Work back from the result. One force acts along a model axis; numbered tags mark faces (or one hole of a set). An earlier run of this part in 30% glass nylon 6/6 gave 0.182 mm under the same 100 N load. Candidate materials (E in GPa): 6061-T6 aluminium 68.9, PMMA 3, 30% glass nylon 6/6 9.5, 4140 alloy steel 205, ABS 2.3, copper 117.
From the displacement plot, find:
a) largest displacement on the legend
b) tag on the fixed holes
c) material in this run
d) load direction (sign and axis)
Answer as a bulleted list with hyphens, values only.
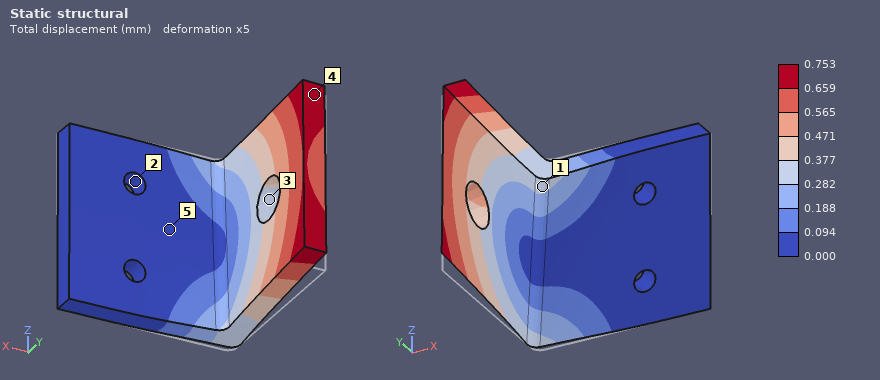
- 0.753 mm
- 2
- ABS
- +Z
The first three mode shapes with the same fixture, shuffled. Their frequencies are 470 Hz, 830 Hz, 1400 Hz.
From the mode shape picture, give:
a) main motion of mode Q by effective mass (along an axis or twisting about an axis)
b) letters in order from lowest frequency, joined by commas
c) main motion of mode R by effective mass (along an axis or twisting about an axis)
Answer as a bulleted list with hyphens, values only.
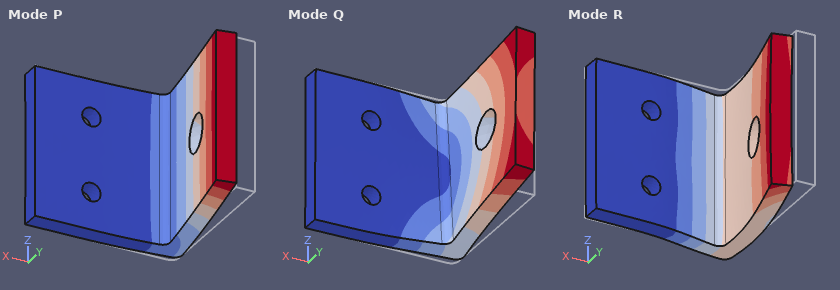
- along Z
- P, Q, R
- along Y
